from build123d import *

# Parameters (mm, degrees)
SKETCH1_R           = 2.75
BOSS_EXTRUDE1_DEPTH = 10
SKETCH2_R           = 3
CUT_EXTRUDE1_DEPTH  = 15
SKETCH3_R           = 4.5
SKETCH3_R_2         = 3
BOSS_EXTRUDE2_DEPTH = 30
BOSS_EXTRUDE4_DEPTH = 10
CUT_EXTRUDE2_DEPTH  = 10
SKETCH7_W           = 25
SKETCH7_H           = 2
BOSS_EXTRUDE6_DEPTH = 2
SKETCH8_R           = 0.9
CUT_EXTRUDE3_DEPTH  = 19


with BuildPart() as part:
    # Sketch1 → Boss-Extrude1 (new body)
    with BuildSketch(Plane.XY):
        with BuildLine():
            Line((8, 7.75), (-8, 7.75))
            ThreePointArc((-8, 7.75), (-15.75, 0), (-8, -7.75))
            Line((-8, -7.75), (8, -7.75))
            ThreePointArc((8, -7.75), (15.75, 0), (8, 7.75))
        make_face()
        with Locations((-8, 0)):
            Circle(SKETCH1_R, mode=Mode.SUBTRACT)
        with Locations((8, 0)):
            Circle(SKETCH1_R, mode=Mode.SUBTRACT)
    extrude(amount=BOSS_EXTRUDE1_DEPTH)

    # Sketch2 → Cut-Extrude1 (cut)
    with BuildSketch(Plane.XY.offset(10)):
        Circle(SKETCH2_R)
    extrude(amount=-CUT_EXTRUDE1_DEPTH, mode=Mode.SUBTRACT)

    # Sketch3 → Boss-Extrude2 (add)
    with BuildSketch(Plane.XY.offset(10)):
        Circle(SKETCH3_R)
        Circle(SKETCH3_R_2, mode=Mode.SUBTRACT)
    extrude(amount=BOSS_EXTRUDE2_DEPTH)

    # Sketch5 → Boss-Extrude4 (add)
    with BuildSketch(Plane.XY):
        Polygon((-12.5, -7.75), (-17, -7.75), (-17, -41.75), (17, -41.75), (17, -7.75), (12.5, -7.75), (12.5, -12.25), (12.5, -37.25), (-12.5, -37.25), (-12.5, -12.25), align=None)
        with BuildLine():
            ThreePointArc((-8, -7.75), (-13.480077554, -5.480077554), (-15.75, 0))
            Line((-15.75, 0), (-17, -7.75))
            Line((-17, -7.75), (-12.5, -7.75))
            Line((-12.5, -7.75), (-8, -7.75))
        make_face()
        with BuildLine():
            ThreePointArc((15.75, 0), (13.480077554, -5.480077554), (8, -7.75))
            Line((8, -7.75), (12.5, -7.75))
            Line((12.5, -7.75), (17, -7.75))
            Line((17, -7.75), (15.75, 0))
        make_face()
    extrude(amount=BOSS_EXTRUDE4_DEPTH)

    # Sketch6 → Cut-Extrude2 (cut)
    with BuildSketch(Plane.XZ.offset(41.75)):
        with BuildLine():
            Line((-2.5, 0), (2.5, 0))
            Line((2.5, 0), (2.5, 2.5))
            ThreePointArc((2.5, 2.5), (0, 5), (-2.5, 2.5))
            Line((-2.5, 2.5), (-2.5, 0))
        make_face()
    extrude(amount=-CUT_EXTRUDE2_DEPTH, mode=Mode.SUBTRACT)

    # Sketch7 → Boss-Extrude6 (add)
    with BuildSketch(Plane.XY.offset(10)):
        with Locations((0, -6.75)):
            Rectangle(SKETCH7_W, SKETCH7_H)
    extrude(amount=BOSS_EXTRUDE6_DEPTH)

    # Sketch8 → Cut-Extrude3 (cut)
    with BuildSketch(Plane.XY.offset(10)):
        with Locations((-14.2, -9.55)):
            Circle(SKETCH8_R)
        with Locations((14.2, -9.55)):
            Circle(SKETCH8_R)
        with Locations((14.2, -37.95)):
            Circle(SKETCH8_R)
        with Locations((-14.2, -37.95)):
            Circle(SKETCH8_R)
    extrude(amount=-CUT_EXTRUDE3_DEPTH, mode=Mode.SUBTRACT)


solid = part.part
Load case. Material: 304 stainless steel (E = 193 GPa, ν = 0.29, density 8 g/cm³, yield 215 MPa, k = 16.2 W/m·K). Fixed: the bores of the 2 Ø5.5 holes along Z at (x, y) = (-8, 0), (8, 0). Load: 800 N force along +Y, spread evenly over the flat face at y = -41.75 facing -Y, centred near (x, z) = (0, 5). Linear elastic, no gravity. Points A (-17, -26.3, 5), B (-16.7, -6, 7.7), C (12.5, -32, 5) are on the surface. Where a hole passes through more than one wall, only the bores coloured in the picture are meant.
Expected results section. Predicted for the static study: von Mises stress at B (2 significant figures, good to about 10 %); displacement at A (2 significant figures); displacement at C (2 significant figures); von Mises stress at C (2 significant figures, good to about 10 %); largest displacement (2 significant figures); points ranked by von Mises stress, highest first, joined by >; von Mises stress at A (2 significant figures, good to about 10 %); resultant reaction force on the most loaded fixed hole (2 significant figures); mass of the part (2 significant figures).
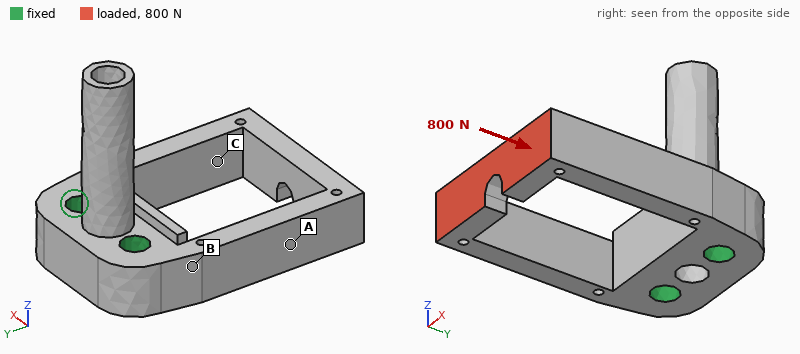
22 MPa
4.7 µm
4.5 µm
33 MPa
12 µm
C > B > A
7.9 MPa
400 N
73 g
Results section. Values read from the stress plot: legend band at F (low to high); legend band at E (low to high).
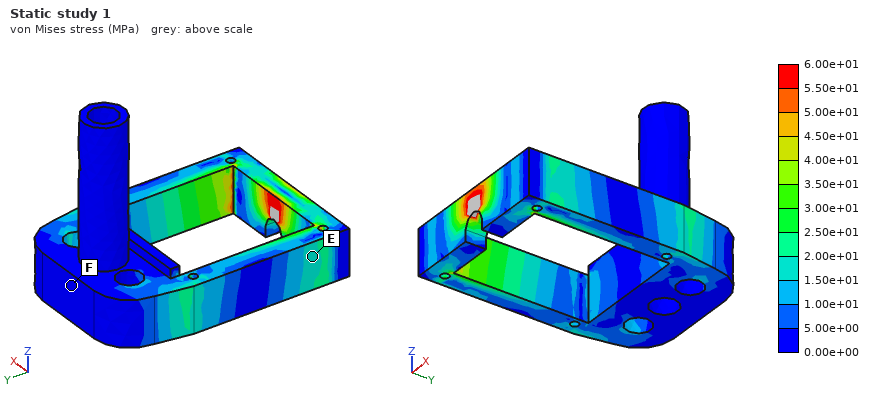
0.00e+00 to 5.00e+00 MPa
1.50e+01 to 2.00e+01 MPa
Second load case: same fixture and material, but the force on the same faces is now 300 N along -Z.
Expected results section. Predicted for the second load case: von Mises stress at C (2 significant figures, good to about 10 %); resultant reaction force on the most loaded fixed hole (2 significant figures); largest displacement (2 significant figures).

13 MPa
150 N
58 µm
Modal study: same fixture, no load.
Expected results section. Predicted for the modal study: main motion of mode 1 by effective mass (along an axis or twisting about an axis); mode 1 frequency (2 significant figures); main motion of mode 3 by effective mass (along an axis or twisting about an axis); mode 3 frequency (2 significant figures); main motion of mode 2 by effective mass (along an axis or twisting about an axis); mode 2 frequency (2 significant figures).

along X
2800 Hz
twisting about Y
5500 Hz
along Z
3200 Hz
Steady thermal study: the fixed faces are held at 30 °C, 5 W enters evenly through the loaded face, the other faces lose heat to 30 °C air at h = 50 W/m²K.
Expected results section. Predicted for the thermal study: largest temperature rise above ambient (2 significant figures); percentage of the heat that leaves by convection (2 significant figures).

61 K
77 %
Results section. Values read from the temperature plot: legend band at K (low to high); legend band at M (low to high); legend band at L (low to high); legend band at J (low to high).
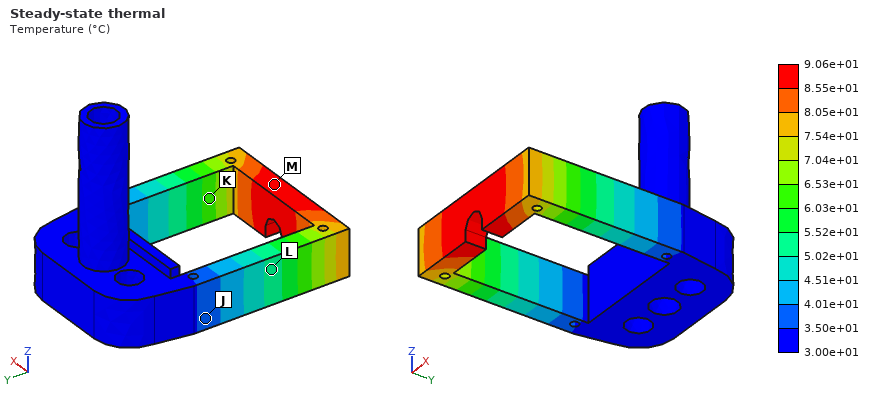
6.03e+01 to 6.53e+01 °C
8.55e+01 to 9.06e+01 °C
5.02e+01 to 5.52e+01 °C
3.50e+01 to 4.01e+01 °C
